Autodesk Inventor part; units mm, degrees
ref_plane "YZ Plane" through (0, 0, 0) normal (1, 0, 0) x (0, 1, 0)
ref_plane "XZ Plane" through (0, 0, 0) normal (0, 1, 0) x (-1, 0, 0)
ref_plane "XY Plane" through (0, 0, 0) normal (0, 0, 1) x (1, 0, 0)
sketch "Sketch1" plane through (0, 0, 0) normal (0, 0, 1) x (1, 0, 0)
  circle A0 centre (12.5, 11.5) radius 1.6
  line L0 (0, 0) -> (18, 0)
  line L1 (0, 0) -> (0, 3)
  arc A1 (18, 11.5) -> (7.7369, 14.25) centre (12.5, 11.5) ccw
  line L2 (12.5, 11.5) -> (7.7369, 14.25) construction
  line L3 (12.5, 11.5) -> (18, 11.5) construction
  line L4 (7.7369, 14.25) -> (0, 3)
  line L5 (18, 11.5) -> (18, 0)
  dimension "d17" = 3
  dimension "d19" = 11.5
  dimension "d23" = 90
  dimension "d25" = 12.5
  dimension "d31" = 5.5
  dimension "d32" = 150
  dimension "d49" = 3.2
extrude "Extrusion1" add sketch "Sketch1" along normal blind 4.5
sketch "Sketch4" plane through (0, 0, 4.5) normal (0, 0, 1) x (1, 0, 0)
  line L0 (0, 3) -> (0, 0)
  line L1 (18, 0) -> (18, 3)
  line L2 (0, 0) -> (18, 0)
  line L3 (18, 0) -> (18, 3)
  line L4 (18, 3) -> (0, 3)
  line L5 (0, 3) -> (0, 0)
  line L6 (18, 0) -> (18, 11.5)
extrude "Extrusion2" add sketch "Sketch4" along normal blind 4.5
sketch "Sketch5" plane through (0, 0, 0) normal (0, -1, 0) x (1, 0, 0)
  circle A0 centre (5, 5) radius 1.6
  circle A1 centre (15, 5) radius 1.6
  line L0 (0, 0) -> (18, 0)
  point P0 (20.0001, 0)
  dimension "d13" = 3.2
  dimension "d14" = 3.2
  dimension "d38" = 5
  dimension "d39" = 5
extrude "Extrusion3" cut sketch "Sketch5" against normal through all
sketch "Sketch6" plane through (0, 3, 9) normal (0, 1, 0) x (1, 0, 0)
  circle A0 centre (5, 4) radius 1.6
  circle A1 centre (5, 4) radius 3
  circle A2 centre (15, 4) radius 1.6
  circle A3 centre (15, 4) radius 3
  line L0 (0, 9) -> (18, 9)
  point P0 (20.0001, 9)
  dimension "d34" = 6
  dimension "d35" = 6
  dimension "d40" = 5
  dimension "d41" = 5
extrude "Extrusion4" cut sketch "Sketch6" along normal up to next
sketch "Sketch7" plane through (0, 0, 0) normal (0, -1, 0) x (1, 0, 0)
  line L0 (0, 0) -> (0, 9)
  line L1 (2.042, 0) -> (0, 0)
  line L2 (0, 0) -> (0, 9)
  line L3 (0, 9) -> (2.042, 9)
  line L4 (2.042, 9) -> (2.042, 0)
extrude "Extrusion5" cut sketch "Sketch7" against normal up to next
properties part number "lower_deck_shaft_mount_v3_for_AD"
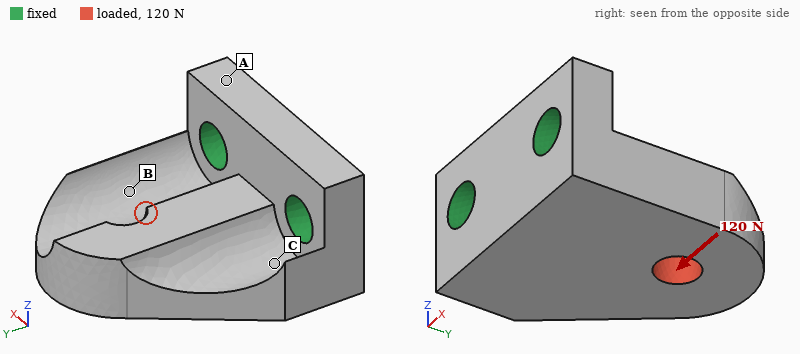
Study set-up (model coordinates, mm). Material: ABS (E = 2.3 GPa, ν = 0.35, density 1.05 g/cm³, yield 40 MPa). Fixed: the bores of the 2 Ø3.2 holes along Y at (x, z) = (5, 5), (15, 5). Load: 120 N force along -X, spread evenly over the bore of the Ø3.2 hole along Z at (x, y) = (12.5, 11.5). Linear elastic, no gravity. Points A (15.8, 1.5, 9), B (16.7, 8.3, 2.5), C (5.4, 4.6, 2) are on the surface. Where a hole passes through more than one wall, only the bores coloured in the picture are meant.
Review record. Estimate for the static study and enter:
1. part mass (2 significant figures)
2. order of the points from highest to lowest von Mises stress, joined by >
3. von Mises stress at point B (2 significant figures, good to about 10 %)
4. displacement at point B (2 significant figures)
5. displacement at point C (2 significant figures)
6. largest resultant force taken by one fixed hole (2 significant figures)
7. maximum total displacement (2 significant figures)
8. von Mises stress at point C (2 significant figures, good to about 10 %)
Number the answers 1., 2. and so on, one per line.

1. 0.96 g
2. C > B > A
3. 6.7 MPa
4. 0.088 mm
5. 0.041 mm
6. 130 N
7. 0.17 mm
8. 13 MPa
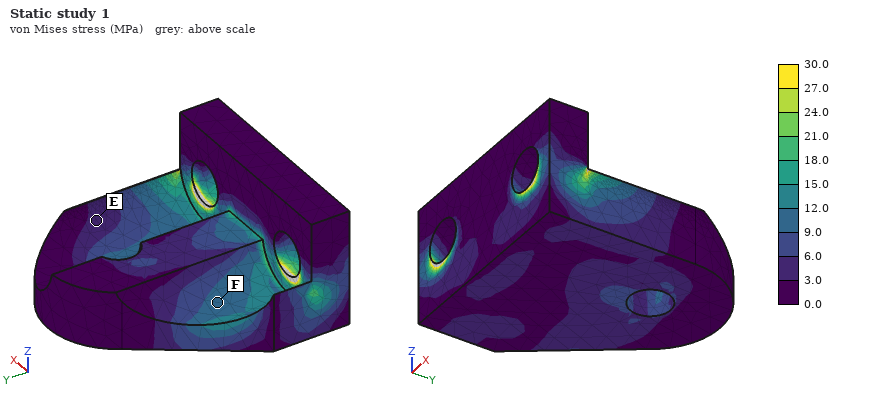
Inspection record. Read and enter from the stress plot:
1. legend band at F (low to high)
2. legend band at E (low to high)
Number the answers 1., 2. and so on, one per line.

1. 9.0 to 12.0 MPa
2. 3.0 to 6.0 MPa
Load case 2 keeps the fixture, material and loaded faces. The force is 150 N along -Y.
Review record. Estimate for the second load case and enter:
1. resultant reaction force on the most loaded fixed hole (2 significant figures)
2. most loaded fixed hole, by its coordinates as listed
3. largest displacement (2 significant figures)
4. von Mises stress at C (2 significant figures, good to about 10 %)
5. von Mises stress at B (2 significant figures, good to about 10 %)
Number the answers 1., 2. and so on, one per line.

1. 100 N
2. (15, 5)
3. 0.12 mm
4. 2.6 MPa
5. 5.3 MPa
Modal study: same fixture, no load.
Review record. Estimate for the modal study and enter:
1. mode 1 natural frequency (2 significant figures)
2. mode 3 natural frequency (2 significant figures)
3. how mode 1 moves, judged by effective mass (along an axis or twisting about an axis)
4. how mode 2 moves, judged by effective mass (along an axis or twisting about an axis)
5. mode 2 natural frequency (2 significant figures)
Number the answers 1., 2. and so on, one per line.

1. 3700 Hz
2. 11 kHz
3. along Z
4. along X
5. 8000 Hz
